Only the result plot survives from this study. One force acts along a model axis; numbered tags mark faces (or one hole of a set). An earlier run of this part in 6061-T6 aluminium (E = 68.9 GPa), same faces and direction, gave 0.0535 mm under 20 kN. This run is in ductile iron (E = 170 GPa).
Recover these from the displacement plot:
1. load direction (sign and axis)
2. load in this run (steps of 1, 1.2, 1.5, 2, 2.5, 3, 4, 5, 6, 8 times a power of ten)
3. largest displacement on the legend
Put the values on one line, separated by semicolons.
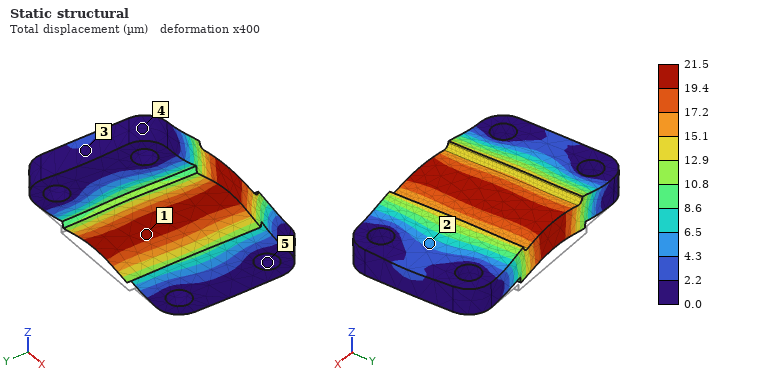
+Z; 20 kN; 21.5 µm
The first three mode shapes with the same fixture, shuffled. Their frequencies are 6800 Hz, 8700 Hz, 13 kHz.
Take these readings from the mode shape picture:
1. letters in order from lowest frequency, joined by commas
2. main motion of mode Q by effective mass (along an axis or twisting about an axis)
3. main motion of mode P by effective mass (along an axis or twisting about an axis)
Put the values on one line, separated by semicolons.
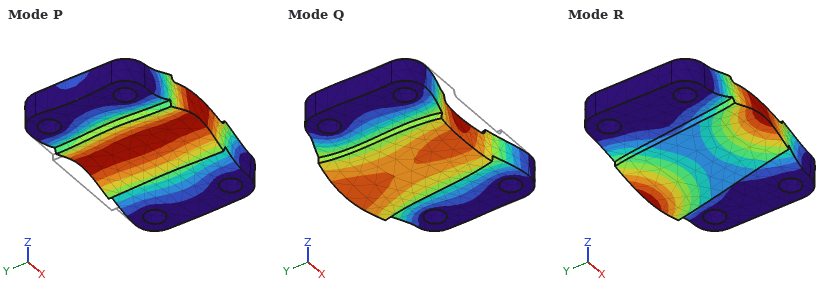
P, R, Q; along Y; along Z
